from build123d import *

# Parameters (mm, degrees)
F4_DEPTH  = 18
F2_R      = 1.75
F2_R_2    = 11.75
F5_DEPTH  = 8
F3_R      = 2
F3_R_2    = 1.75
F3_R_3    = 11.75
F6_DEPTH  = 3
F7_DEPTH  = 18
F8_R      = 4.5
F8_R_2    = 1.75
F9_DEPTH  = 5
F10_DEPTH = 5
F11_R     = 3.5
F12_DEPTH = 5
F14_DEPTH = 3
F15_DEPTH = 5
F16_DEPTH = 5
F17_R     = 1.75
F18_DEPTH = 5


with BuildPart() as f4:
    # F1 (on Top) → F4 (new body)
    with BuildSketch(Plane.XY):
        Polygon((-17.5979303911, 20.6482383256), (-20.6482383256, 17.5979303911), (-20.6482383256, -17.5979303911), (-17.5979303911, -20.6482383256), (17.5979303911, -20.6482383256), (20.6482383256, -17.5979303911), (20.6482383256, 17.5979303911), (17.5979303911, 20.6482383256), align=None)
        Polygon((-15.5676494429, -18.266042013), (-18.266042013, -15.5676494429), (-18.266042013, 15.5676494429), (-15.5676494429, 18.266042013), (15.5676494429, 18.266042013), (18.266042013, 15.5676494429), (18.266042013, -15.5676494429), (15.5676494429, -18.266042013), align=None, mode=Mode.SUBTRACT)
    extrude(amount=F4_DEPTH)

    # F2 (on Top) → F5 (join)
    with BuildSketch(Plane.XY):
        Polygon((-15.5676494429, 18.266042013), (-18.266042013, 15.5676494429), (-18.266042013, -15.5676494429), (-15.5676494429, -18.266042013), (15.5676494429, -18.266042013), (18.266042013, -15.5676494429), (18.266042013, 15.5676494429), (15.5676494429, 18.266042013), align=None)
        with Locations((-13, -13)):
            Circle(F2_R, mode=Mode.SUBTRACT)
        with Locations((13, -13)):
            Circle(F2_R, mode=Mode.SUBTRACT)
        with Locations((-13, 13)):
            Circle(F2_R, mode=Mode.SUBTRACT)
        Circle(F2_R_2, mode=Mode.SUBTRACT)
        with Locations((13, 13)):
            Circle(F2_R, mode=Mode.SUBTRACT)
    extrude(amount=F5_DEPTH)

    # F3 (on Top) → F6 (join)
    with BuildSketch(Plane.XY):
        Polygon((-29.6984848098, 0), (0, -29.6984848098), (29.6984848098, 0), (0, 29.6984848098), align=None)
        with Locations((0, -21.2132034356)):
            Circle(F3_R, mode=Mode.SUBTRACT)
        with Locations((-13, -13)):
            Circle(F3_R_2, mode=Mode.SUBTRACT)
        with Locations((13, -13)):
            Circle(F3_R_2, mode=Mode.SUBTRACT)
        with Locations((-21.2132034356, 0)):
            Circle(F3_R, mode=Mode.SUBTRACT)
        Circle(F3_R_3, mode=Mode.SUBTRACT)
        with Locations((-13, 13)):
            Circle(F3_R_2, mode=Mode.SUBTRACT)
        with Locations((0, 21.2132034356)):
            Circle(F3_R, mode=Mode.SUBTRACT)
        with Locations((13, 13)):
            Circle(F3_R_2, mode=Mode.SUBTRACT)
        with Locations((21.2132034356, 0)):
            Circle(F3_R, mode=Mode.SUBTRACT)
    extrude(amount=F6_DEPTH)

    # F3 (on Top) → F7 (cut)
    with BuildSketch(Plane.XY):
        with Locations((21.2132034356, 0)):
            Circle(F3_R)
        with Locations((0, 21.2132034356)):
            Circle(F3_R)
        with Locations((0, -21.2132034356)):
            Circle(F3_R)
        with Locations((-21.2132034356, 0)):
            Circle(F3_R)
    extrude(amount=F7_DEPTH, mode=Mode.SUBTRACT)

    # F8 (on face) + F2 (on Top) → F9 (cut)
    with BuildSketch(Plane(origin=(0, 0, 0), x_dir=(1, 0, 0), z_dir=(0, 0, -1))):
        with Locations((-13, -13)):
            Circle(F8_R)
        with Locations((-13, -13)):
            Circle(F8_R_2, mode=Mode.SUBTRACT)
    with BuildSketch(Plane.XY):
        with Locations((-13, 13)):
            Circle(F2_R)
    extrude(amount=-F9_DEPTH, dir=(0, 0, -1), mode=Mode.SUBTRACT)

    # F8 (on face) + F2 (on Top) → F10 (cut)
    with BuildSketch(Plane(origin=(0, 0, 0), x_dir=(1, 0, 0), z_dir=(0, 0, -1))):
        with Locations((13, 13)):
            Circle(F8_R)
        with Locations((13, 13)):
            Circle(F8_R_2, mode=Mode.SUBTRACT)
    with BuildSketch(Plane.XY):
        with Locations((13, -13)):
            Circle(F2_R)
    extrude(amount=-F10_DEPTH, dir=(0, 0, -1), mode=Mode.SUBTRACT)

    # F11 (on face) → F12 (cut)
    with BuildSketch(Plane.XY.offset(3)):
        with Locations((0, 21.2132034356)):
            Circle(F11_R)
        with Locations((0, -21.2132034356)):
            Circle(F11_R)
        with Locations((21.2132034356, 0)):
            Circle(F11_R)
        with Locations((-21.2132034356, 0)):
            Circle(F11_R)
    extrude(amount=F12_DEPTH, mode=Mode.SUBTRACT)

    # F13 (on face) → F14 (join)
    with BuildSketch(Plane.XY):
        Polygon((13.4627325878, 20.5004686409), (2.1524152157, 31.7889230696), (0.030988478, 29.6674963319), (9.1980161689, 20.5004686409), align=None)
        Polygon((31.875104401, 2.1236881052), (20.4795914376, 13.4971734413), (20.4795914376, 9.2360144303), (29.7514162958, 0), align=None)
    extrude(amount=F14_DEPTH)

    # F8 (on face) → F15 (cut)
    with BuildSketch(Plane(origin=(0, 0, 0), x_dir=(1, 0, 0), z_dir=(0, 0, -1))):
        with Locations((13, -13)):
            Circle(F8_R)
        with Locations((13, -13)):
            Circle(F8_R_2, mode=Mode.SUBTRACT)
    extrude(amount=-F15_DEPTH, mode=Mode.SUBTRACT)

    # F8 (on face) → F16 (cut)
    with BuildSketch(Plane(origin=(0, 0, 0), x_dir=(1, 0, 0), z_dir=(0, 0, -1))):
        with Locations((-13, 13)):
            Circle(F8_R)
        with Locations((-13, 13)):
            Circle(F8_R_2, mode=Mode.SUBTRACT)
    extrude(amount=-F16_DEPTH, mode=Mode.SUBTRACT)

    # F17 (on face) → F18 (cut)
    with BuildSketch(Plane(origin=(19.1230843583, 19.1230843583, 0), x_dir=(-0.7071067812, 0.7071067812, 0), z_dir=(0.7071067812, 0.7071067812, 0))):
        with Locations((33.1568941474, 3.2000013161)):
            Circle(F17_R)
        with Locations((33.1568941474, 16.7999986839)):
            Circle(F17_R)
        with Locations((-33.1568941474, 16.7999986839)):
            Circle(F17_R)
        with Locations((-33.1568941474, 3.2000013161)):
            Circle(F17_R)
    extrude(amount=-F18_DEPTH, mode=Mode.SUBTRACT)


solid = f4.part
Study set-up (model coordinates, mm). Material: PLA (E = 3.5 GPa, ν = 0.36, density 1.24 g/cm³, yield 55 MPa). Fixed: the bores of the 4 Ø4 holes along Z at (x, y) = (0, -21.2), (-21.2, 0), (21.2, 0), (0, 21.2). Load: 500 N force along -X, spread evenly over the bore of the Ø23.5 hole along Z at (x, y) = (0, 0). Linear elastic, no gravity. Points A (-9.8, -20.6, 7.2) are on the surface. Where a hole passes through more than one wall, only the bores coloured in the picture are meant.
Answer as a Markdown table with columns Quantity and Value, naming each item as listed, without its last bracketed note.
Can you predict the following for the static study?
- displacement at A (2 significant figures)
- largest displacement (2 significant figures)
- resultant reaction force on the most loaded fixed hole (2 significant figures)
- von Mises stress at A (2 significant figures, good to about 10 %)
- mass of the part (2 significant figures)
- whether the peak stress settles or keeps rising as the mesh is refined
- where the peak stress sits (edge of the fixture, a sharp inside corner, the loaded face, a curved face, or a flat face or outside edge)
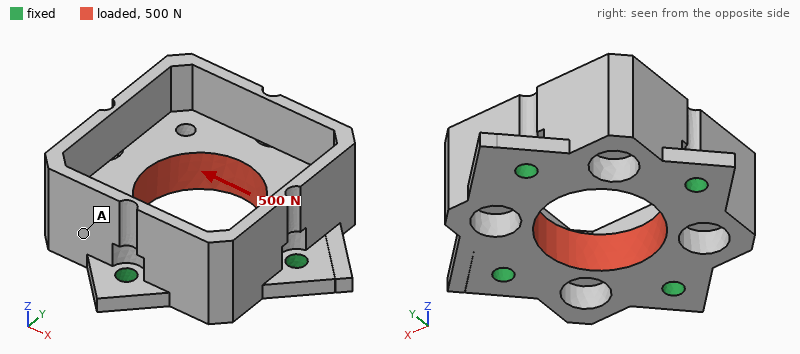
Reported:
| Quantity | Value |
|---|---|
| displacement at A | 10 µm |
| largest displacement | 20 µm |
| resultant reaction force on the most loaded fixed hole | 140 N |
| von Mises stress at A | 1.2 MPa |
| mass of the part | 16 g |
| whether the peak stress settles or keeps rising as the mesh is refined | keeps rising |
| where the peak stress sits | edge of the fixture |
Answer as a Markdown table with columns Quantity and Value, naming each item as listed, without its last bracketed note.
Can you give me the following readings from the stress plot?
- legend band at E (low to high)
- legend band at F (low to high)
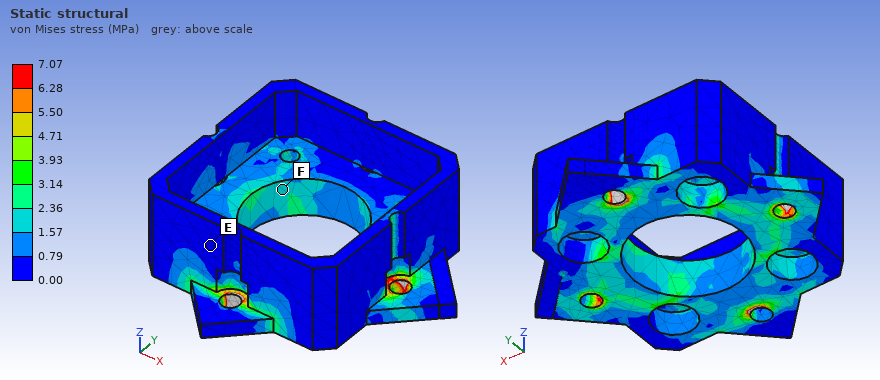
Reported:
| Quantity | Value |
|---|---|
| legend band at E | 0.00 to 0.79 MPa |
| legend band at F | 1.57 to 2.36 MPa |
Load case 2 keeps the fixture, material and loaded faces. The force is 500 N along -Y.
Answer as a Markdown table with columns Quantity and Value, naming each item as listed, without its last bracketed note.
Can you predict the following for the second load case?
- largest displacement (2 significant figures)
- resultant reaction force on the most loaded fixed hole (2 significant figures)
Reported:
| Quantity | Value |
|---|---|
| largest displacement | 20 µm |
| resultant reaction force on the most loaded fixed hole | 140 N |
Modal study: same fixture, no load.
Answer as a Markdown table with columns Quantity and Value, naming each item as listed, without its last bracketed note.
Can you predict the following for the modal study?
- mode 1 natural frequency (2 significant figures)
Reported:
| Quantity | Value |
|---|---|
| mode 1 natural frequency | 3500 Hz |
